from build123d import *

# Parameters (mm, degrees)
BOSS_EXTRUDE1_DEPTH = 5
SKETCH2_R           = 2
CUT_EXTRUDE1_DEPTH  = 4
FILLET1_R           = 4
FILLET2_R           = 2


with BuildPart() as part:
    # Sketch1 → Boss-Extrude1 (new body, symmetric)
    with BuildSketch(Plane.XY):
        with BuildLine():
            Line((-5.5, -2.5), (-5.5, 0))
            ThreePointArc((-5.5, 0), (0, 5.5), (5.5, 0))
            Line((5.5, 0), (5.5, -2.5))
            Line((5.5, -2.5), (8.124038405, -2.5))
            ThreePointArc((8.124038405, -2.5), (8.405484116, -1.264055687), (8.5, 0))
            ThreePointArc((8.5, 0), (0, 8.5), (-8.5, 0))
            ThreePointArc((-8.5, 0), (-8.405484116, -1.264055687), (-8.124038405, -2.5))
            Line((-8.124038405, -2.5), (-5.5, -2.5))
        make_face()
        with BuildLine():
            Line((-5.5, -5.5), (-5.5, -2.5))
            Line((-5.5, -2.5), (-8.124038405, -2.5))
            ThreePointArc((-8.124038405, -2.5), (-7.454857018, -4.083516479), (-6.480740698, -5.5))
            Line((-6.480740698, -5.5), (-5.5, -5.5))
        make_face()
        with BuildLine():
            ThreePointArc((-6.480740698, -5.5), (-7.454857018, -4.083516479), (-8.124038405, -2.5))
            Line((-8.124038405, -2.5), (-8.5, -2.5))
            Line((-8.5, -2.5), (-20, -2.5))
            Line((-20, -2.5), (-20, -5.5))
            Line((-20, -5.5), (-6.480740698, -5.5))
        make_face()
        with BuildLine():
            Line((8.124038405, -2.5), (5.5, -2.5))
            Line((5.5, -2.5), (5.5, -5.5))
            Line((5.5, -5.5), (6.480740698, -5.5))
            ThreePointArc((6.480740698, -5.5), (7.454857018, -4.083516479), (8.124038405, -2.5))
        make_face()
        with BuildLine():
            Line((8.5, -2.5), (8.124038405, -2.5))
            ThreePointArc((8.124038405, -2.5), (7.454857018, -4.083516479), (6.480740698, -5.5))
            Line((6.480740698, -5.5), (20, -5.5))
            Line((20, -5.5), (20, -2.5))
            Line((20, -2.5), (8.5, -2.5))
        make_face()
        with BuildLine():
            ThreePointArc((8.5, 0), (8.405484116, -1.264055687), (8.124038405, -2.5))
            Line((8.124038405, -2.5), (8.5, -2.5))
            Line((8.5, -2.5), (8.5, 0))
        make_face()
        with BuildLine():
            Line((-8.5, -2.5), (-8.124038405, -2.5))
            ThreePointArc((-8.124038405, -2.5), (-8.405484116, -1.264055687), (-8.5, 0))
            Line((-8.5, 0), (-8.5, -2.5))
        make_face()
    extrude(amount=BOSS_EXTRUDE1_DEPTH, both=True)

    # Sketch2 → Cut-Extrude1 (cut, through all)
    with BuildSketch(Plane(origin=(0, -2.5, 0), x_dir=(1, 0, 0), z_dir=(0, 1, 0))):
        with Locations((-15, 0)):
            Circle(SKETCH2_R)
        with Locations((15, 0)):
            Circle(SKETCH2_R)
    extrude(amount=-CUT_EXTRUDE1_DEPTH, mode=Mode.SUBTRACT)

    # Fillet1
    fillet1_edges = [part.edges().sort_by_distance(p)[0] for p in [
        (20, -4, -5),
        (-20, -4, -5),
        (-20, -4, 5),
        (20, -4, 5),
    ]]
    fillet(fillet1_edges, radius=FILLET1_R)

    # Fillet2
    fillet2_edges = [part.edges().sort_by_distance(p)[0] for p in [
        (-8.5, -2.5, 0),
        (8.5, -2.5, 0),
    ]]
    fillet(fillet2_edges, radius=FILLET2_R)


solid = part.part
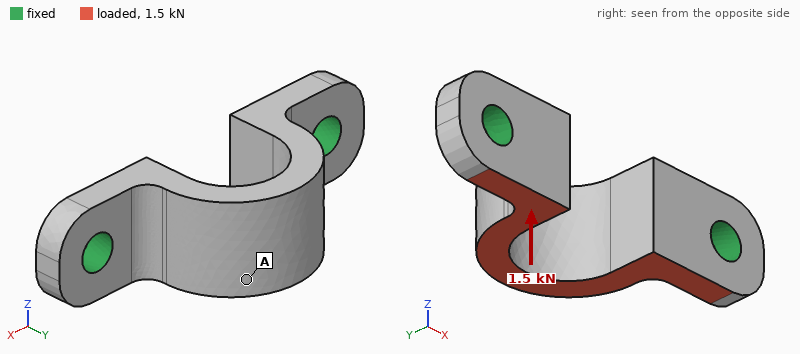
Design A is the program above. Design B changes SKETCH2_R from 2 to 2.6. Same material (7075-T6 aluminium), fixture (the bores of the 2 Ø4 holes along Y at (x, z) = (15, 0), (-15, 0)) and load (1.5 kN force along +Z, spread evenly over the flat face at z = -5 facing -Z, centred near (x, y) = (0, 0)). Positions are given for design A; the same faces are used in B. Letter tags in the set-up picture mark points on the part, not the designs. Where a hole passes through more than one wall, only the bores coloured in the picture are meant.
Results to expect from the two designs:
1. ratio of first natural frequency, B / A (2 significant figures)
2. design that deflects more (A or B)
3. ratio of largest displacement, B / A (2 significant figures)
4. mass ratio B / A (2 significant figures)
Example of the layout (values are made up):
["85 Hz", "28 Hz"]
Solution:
["1.1", "A", "0.80", "0.97"]
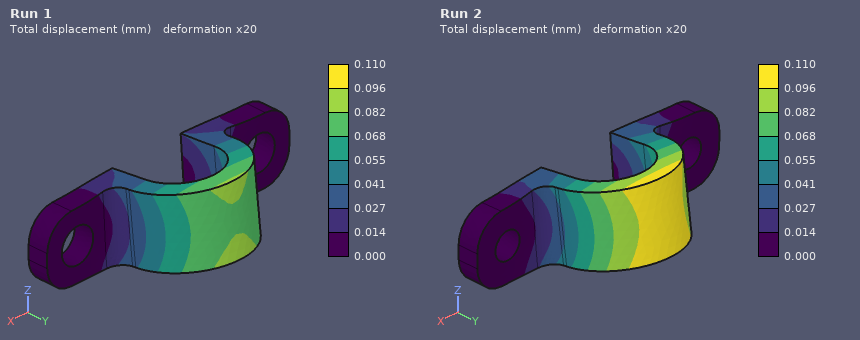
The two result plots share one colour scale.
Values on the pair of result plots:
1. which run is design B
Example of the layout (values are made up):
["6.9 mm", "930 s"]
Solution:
["Run 1"]
